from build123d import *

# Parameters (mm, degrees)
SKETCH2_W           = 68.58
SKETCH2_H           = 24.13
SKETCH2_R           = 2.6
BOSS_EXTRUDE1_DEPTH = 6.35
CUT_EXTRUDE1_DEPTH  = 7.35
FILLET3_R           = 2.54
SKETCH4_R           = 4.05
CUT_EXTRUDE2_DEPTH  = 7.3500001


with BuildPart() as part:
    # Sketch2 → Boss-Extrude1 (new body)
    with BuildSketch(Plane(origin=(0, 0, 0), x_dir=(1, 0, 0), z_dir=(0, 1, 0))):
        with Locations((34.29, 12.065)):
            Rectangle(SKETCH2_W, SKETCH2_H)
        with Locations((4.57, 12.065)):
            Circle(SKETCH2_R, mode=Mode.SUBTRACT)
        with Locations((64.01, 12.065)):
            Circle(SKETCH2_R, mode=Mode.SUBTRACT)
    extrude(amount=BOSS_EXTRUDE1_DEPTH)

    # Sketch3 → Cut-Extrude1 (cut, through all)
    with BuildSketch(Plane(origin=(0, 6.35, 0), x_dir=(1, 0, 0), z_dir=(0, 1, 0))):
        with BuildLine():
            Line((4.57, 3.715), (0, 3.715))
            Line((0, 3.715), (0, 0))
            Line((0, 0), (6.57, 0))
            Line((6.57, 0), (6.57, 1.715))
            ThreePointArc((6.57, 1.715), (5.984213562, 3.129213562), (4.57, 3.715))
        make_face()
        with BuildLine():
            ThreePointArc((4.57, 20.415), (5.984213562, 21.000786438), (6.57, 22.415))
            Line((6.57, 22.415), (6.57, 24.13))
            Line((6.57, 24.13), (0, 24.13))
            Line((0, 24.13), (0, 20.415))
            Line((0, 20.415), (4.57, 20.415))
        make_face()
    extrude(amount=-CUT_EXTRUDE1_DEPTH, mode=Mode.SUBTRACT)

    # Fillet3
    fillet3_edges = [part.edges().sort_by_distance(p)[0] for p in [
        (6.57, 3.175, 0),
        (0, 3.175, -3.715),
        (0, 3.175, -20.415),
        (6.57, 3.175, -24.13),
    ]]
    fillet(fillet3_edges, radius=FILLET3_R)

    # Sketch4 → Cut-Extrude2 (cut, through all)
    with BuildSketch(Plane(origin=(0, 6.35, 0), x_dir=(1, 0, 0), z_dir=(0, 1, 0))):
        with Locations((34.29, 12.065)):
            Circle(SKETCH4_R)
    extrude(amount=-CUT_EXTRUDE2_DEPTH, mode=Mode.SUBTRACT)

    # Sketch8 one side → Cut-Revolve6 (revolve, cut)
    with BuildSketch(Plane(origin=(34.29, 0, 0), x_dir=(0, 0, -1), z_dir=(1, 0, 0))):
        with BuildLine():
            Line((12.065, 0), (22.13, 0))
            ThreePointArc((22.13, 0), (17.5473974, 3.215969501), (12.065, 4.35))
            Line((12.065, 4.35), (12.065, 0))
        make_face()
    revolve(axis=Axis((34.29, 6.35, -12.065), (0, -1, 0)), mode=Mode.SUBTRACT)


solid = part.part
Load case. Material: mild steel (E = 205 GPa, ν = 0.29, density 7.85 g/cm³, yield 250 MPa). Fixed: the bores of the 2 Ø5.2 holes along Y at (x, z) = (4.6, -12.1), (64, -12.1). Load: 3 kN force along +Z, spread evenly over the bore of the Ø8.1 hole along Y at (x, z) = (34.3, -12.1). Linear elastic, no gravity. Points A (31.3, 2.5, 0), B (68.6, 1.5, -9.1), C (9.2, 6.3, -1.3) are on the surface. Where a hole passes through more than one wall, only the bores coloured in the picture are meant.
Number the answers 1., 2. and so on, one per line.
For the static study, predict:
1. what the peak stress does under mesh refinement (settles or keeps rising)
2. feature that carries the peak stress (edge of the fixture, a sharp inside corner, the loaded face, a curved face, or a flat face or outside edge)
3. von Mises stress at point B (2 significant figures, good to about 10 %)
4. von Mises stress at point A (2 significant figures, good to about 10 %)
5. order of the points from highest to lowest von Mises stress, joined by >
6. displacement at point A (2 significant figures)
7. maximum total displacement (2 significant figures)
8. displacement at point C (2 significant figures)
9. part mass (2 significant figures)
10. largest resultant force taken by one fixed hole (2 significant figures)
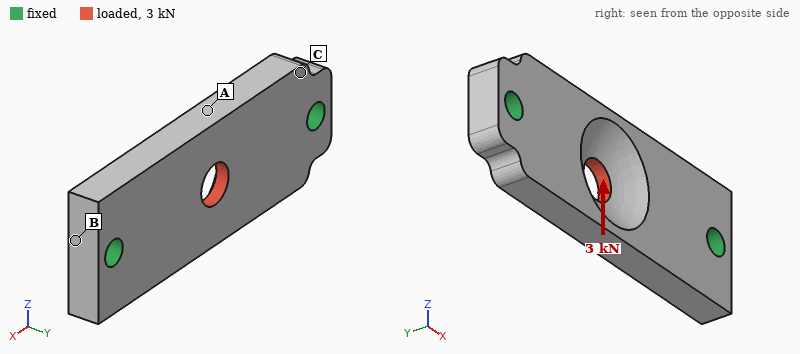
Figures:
1. keeps rising
2. edge of the fixture
3. 29 MPa
4. 62 MPa
5. A > B > C
6. 11 µm
7. 13 µm
8. 3.8 µm
9. 71 g
10. 1.5 kN
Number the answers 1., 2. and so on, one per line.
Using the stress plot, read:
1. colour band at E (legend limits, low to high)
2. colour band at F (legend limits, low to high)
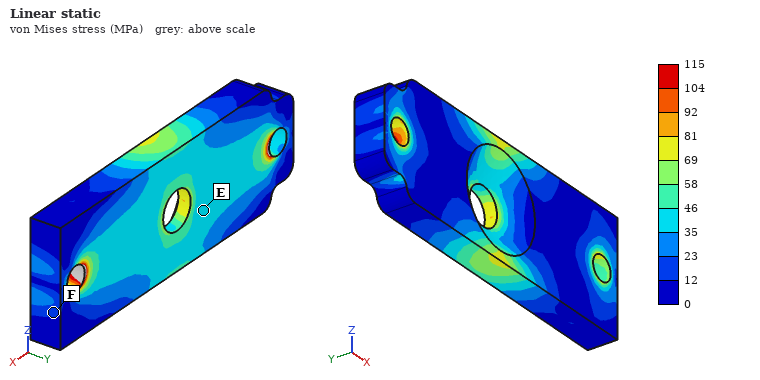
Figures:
1. 35 to 46 MPa
2. 12 to 23 MPa
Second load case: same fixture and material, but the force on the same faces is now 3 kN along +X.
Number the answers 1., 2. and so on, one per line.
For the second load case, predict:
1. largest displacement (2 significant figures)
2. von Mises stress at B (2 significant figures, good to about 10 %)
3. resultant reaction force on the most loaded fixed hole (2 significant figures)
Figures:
1. 2.9 µm
2. 11 MPa
3. 1.5 kN
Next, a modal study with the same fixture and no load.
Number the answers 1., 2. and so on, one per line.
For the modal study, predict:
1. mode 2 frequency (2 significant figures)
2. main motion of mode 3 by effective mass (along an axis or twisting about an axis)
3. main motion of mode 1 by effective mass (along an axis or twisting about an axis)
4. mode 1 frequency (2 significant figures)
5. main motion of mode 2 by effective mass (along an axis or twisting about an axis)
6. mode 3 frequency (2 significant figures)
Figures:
1. 12 kHz
2. along Z
3. along Y
4. 8500 Hz
5. twisting about X
6. 17 kHz
